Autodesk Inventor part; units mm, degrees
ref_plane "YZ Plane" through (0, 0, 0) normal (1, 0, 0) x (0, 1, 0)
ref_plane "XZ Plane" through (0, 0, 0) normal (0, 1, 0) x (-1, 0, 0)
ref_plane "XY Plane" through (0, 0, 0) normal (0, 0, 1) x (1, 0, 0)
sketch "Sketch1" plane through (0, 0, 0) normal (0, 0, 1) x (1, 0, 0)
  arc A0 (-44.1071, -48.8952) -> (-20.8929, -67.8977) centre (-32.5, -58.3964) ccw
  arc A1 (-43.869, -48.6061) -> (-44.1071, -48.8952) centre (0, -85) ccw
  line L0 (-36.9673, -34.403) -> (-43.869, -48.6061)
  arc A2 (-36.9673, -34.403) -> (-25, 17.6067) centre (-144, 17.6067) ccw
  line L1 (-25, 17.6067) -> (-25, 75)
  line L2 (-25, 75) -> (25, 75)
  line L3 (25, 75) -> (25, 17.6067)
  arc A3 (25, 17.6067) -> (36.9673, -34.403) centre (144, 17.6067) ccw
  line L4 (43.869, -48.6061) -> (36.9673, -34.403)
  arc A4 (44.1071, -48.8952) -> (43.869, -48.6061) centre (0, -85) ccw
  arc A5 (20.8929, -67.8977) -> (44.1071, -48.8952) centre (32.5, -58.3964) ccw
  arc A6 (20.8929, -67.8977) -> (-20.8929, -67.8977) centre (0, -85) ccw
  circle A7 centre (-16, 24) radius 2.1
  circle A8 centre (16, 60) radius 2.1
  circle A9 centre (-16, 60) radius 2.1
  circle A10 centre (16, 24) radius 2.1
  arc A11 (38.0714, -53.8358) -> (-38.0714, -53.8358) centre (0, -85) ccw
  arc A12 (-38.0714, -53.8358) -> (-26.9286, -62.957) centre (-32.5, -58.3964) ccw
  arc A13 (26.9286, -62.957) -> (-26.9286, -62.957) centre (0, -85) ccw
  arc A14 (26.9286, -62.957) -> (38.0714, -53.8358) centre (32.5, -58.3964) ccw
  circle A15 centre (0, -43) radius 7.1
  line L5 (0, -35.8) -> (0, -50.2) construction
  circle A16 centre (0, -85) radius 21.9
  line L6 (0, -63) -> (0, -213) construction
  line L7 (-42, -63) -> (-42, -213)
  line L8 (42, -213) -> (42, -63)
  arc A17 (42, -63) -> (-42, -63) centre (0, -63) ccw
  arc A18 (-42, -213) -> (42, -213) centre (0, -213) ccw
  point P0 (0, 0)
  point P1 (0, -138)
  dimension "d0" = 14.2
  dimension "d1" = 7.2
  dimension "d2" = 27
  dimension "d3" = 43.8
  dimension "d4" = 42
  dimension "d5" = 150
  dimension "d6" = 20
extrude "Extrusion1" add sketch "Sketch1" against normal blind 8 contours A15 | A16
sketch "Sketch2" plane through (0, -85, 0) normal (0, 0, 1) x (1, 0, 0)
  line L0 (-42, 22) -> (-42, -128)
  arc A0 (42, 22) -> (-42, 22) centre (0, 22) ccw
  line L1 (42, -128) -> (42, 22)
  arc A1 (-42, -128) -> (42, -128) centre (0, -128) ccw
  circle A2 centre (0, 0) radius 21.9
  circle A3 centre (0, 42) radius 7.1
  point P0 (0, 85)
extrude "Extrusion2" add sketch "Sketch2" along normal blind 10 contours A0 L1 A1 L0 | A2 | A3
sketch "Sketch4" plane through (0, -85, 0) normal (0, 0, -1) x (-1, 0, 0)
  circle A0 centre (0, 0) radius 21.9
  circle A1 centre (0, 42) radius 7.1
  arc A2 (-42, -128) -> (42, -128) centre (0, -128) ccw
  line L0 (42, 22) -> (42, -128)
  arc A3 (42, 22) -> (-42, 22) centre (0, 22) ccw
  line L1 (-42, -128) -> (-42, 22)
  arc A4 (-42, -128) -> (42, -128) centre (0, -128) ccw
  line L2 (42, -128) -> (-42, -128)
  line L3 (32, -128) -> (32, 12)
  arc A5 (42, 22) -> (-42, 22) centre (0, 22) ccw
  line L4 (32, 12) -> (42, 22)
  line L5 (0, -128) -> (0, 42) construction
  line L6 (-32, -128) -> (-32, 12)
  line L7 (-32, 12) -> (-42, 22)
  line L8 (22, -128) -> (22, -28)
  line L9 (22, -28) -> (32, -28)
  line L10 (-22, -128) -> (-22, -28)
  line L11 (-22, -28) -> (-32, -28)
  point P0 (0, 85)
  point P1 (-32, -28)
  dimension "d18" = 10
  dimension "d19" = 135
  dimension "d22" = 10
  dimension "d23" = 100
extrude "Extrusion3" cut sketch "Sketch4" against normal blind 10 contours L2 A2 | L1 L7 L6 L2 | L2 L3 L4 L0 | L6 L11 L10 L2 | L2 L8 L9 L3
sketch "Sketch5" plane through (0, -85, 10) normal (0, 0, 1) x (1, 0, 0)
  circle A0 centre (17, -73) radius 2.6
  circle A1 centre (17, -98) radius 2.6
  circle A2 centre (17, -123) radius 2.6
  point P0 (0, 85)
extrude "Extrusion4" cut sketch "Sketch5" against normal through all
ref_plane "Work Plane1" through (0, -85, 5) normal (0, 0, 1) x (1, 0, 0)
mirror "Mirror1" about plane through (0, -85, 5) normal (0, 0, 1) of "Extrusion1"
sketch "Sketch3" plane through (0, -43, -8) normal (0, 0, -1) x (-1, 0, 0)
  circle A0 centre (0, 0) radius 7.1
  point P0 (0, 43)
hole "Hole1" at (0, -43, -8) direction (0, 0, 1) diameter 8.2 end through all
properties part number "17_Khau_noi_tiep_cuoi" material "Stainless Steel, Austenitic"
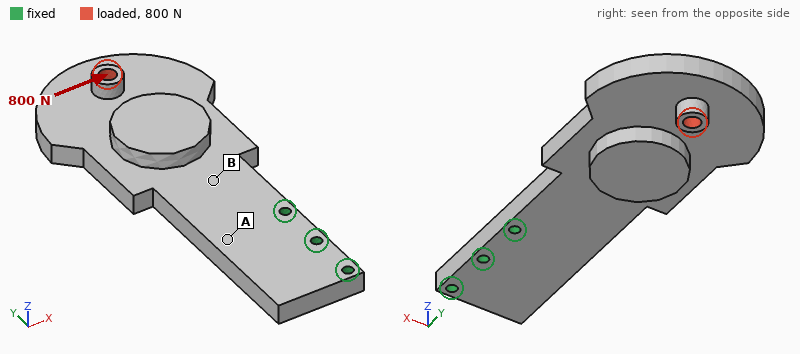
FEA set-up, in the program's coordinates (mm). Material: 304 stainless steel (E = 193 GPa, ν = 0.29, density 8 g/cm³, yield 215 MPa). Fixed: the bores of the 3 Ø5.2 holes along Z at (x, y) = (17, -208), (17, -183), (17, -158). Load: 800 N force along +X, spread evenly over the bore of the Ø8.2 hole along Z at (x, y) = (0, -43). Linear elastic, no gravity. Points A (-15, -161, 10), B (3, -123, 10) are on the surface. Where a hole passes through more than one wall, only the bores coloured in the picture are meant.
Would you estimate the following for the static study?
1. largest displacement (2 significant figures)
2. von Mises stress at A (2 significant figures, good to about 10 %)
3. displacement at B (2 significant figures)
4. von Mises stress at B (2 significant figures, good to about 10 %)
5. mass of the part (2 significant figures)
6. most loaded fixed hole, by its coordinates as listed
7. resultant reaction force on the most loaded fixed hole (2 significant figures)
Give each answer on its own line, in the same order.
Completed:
53 µm
15 MPa
9.8 µm
5.6 MPa
1.0 kg
(17, -158)
3.3 kN
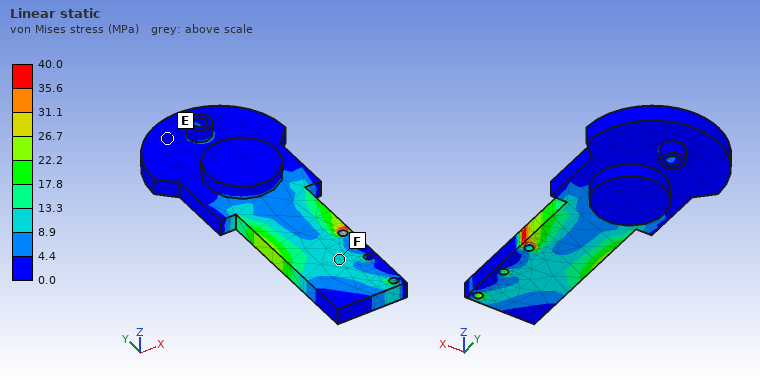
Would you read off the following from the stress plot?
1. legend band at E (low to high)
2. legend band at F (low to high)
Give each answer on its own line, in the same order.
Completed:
0.0 to 4.4 MPa
8.9 to 13.3 MPa
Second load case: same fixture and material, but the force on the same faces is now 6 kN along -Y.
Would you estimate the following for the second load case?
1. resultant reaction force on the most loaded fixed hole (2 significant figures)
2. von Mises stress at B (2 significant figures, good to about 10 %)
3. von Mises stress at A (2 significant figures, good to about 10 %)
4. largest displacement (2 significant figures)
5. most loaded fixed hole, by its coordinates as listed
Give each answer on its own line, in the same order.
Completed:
3.8 kN
13 MPa
14 MPa
22 µm
(17, -158)
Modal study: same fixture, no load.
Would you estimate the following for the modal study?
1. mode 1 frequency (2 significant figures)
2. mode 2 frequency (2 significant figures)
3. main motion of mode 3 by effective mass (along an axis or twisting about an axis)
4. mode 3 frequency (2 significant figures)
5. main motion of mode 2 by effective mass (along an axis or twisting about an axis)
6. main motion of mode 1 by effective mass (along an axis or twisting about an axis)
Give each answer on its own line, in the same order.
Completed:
300 Hz
1100 Hz
twisting about Y
1200 Hz
along X
along Z
